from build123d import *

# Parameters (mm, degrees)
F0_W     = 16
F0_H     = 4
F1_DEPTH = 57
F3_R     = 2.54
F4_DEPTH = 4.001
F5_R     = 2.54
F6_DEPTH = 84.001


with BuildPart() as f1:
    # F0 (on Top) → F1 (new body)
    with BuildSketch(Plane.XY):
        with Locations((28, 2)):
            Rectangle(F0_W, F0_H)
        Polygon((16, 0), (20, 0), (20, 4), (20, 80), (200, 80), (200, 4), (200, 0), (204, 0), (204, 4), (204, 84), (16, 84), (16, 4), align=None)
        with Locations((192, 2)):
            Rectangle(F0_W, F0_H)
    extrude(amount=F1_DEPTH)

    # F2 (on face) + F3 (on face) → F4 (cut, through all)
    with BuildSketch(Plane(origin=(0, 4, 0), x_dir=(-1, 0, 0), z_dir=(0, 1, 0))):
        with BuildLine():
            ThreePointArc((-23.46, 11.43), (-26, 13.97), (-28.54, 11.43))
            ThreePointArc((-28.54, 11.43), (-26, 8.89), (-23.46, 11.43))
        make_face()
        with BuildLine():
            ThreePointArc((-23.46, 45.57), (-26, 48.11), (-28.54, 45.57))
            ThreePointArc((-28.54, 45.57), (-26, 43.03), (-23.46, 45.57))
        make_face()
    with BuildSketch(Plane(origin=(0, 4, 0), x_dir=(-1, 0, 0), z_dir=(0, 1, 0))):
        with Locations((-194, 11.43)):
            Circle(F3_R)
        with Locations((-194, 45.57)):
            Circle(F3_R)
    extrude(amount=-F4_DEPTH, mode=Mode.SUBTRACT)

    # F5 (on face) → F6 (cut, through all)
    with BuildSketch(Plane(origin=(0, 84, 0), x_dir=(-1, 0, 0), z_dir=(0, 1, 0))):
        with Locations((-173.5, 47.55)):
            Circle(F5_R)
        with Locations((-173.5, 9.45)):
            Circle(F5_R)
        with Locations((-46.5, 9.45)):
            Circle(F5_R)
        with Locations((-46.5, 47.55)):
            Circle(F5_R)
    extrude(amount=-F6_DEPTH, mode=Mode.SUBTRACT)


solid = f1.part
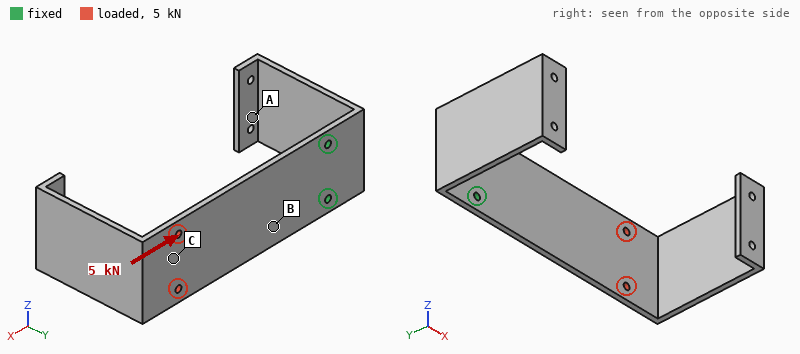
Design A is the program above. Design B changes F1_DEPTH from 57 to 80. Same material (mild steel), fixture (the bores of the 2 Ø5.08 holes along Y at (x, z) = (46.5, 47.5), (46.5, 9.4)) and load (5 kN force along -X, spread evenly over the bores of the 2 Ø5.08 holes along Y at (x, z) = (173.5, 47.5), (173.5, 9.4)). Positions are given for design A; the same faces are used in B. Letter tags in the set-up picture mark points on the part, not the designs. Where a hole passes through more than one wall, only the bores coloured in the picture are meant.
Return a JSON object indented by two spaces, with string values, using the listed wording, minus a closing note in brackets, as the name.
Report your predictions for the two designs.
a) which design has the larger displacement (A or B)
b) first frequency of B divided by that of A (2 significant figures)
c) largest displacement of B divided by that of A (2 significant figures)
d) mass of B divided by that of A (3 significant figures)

{
  "which design has the larger displacement": "B",
  "first frequency of B divided by that of A": "0.99",
  "largest displacement of B divided by that of A": "1.6",
  "mass of B divided by that of A": "1.41"
}
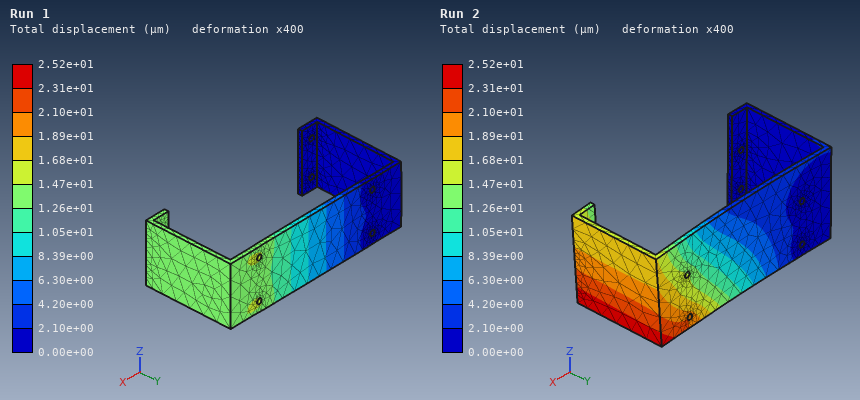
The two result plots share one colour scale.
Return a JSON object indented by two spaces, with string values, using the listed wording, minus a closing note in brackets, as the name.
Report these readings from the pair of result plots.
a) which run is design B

{
  "which run is design B": "Run 2"
}
